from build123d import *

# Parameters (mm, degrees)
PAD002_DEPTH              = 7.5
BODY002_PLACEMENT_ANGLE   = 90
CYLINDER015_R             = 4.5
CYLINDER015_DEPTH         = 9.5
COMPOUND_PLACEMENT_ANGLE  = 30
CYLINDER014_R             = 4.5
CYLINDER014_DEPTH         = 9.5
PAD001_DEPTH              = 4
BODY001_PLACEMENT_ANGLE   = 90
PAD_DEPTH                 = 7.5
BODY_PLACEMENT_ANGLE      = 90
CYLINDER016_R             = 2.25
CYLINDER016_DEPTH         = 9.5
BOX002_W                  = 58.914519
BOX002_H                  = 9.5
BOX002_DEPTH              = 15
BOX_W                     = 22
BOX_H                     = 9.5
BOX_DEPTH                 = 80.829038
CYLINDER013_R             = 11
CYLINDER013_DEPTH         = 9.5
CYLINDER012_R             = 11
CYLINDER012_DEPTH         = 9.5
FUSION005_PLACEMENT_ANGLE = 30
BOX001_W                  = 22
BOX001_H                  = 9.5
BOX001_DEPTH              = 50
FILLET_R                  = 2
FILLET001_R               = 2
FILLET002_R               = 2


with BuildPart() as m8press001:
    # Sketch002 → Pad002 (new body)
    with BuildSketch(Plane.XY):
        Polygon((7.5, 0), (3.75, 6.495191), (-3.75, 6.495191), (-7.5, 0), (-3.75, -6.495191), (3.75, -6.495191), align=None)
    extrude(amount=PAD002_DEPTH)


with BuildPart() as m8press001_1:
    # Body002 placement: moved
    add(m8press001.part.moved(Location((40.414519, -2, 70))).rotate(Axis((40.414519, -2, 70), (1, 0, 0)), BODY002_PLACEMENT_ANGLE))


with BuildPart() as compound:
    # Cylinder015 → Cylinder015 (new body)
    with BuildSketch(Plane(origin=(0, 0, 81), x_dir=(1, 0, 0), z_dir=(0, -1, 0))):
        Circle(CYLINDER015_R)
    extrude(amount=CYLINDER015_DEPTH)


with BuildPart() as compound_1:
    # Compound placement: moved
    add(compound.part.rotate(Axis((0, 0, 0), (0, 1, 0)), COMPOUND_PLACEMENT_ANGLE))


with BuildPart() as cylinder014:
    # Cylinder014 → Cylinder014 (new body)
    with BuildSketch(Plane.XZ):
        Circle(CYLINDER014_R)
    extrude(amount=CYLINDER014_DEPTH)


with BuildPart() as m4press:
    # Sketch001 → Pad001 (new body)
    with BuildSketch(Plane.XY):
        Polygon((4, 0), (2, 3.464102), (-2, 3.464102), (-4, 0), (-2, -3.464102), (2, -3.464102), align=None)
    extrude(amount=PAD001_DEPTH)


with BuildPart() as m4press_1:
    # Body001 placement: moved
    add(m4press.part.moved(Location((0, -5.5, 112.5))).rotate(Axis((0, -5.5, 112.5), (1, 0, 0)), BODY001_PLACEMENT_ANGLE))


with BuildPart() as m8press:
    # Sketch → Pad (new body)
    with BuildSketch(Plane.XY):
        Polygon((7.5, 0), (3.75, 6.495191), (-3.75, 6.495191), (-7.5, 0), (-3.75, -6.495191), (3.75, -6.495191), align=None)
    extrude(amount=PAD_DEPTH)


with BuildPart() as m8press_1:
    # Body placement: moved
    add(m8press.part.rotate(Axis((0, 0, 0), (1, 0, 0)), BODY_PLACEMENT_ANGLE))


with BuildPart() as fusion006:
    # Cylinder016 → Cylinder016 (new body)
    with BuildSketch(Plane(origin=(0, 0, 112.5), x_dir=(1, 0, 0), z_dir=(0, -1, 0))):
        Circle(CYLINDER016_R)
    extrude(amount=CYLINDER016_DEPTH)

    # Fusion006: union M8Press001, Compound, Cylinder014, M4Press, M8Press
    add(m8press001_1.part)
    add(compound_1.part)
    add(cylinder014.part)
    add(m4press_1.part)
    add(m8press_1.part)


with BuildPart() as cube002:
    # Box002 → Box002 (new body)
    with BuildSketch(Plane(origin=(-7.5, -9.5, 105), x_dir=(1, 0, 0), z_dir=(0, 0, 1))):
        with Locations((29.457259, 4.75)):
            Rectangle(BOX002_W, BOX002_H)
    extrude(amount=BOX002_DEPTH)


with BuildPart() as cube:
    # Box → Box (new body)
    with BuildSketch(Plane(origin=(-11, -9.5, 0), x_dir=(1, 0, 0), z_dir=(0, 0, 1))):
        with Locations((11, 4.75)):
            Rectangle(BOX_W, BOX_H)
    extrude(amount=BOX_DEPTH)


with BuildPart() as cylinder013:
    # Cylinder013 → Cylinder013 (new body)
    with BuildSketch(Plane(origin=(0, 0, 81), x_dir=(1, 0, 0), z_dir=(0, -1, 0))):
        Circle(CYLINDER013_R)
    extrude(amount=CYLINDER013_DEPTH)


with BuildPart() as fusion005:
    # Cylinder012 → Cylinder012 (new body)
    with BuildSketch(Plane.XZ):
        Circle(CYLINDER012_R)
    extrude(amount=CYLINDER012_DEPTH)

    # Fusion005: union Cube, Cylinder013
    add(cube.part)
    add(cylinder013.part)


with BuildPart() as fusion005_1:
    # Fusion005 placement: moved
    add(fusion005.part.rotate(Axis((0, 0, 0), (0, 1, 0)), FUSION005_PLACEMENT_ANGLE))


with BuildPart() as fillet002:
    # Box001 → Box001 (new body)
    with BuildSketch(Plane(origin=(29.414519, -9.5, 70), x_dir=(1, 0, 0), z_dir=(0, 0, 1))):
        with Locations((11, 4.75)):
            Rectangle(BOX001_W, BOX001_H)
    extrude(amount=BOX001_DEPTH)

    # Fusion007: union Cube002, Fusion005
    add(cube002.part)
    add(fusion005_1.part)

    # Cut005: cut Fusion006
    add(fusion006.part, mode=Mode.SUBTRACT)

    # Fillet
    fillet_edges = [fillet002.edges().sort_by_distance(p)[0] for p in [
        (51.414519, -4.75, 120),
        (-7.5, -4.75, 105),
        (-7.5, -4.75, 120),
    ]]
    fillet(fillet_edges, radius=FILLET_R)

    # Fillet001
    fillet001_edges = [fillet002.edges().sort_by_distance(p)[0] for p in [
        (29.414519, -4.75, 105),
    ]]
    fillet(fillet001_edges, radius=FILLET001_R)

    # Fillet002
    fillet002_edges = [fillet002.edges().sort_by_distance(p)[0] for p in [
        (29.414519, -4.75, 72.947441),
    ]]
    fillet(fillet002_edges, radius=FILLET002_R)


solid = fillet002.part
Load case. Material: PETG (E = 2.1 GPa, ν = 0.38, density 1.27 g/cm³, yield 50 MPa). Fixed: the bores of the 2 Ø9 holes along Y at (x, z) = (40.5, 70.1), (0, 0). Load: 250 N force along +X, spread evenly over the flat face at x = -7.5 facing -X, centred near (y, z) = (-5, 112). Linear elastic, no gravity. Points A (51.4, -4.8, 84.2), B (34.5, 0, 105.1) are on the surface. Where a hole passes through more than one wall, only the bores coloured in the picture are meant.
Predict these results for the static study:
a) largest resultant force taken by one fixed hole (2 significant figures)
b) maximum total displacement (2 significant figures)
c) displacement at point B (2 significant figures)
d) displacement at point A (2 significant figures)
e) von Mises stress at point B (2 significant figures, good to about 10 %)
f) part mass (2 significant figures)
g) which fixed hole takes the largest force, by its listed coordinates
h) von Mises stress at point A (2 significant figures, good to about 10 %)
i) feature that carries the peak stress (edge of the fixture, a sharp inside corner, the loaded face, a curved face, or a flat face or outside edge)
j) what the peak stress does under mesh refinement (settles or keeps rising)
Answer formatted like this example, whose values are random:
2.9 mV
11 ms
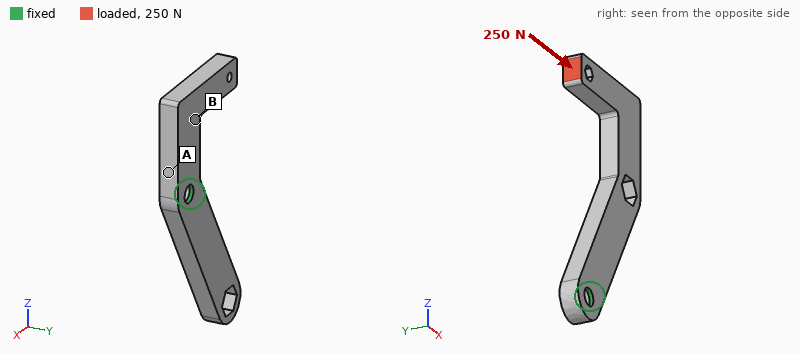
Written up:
300 N
1.6 mm
0.71 mm
0.32 mm
3.2 MPa
40 g
(40.5, 70.1)
10 MPa
edge of the fixture
keeps rising
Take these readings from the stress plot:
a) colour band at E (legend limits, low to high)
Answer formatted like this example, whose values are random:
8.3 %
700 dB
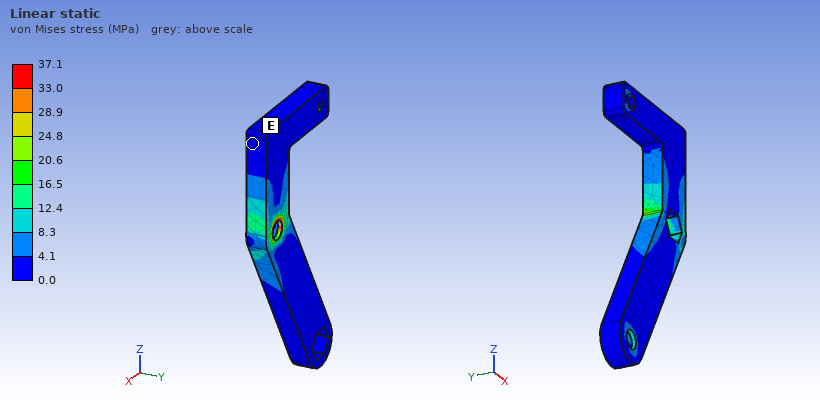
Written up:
0.0 to 4.1 MPa
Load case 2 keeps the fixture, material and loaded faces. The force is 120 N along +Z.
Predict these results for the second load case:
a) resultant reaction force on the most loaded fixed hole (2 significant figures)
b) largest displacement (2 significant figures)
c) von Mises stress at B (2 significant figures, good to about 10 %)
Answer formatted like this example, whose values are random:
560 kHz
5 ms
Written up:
64 N
1.7 mm
3.7 MPa
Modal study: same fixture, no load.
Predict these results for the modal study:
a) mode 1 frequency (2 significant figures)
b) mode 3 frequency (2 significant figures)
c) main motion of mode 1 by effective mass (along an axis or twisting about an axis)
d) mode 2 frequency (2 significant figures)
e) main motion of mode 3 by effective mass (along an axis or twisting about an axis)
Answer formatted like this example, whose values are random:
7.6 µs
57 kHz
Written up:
300 Hz
700 Hz
along Y
640 Hz
twisting about Z
